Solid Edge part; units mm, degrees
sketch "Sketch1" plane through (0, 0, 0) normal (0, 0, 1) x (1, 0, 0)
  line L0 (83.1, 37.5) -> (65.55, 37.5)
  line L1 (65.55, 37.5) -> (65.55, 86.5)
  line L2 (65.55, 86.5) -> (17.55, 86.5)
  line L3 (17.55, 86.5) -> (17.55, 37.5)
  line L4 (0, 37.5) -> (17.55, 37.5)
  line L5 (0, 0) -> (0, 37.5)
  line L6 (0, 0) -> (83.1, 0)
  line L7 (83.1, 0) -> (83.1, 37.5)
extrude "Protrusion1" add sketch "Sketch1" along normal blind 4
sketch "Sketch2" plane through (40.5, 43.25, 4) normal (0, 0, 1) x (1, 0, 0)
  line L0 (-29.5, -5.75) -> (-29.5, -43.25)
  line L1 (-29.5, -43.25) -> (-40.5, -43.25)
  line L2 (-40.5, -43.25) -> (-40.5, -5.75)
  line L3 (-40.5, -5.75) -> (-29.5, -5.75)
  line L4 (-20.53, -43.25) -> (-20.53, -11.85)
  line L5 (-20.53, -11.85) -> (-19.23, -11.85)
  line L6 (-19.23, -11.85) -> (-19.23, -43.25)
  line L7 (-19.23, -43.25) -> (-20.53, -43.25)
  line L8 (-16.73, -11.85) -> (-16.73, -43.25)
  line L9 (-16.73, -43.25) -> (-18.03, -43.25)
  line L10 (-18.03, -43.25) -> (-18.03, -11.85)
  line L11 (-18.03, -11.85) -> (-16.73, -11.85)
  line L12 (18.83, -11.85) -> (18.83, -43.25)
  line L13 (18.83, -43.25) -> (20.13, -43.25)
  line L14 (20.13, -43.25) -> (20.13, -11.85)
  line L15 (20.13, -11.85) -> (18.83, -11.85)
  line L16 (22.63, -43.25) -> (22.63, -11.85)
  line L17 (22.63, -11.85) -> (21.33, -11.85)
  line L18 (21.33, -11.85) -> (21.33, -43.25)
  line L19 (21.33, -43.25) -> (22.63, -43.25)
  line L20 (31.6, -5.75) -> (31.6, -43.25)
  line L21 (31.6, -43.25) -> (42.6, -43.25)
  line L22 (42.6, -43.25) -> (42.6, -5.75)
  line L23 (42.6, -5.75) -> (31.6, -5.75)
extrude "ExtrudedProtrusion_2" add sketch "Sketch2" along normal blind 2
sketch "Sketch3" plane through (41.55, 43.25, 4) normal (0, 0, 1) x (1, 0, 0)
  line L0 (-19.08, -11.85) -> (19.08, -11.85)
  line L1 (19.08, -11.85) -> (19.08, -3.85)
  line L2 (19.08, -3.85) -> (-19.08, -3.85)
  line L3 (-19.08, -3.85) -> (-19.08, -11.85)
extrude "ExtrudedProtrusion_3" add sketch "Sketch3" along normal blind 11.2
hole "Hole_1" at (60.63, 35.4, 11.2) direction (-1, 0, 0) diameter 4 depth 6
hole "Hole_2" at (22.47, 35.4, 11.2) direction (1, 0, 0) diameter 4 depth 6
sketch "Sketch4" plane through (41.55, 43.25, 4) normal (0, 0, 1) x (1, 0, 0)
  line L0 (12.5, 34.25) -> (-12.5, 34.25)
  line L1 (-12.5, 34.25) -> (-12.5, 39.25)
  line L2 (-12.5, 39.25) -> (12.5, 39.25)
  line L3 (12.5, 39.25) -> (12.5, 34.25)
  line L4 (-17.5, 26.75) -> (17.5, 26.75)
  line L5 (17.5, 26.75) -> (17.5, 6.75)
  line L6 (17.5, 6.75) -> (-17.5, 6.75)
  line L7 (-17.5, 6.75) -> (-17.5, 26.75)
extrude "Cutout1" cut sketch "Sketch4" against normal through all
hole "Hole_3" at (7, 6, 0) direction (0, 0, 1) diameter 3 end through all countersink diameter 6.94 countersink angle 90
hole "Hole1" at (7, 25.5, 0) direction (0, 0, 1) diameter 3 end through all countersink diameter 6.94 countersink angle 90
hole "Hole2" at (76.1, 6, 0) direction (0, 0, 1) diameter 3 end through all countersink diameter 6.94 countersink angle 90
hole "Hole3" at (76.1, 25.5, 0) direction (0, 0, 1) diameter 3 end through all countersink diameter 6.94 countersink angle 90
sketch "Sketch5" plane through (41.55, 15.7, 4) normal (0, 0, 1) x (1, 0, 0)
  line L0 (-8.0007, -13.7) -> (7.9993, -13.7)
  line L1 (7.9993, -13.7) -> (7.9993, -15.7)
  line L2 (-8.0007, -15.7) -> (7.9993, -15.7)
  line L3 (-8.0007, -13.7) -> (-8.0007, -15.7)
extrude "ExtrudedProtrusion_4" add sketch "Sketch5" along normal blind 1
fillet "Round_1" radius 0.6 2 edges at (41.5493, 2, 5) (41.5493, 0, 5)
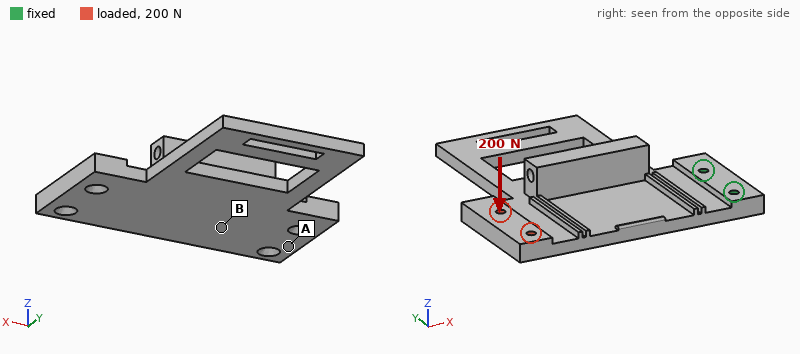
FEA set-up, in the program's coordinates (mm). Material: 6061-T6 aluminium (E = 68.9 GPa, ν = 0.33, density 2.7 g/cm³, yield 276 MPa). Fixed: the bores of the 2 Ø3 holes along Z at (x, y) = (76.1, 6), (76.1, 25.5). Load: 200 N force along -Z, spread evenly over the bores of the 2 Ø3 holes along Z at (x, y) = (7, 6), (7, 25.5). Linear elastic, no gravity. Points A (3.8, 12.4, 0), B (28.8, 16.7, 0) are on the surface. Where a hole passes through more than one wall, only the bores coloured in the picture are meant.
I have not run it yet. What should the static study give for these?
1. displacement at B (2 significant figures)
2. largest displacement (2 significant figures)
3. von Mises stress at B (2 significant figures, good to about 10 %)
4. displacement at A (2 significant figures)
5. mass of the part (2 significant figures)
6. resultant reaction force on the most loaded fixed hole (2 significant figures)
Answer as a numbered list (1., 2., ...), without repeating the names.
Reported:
1. 0.67 mm
2. 1.3 mm
3. 28 MPa
4. 1.2 mm
5. 64 g
6. 160 N
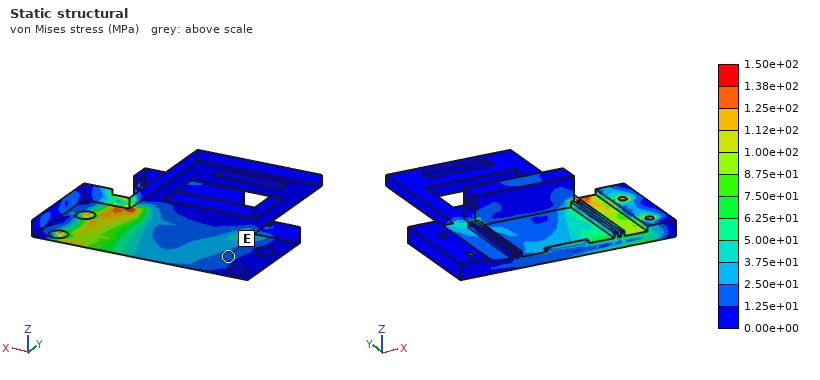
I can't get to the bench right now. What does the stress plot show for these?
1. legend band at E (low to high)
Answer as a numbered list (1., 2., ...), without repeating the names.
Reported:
1. 1.25e+01 to 2.50e+01 MPa
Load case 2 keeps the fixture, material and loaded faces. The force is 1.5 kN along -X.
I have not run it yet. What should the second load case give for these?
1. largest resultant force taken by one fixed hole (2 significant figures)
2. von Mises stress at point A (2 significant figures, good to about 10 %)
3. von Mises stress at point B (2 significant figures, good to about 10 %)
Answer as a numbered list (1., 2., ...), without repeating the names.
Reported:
1. 760 N
2. 3.6 MPa
3. 9.5 MPa
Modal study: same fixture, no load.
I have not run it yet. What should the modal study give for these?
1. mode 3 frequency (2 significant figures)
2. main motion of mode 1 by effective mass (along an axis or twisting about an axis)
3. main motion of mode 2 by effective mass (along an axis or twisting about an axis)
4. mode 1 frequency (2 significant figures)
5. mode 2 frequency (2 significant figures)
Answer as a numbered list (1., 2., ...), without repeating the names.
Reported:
1. 2100 Hz
2. along Z
3. twisting about X
4. 460 Hz
5. 780 Hz
